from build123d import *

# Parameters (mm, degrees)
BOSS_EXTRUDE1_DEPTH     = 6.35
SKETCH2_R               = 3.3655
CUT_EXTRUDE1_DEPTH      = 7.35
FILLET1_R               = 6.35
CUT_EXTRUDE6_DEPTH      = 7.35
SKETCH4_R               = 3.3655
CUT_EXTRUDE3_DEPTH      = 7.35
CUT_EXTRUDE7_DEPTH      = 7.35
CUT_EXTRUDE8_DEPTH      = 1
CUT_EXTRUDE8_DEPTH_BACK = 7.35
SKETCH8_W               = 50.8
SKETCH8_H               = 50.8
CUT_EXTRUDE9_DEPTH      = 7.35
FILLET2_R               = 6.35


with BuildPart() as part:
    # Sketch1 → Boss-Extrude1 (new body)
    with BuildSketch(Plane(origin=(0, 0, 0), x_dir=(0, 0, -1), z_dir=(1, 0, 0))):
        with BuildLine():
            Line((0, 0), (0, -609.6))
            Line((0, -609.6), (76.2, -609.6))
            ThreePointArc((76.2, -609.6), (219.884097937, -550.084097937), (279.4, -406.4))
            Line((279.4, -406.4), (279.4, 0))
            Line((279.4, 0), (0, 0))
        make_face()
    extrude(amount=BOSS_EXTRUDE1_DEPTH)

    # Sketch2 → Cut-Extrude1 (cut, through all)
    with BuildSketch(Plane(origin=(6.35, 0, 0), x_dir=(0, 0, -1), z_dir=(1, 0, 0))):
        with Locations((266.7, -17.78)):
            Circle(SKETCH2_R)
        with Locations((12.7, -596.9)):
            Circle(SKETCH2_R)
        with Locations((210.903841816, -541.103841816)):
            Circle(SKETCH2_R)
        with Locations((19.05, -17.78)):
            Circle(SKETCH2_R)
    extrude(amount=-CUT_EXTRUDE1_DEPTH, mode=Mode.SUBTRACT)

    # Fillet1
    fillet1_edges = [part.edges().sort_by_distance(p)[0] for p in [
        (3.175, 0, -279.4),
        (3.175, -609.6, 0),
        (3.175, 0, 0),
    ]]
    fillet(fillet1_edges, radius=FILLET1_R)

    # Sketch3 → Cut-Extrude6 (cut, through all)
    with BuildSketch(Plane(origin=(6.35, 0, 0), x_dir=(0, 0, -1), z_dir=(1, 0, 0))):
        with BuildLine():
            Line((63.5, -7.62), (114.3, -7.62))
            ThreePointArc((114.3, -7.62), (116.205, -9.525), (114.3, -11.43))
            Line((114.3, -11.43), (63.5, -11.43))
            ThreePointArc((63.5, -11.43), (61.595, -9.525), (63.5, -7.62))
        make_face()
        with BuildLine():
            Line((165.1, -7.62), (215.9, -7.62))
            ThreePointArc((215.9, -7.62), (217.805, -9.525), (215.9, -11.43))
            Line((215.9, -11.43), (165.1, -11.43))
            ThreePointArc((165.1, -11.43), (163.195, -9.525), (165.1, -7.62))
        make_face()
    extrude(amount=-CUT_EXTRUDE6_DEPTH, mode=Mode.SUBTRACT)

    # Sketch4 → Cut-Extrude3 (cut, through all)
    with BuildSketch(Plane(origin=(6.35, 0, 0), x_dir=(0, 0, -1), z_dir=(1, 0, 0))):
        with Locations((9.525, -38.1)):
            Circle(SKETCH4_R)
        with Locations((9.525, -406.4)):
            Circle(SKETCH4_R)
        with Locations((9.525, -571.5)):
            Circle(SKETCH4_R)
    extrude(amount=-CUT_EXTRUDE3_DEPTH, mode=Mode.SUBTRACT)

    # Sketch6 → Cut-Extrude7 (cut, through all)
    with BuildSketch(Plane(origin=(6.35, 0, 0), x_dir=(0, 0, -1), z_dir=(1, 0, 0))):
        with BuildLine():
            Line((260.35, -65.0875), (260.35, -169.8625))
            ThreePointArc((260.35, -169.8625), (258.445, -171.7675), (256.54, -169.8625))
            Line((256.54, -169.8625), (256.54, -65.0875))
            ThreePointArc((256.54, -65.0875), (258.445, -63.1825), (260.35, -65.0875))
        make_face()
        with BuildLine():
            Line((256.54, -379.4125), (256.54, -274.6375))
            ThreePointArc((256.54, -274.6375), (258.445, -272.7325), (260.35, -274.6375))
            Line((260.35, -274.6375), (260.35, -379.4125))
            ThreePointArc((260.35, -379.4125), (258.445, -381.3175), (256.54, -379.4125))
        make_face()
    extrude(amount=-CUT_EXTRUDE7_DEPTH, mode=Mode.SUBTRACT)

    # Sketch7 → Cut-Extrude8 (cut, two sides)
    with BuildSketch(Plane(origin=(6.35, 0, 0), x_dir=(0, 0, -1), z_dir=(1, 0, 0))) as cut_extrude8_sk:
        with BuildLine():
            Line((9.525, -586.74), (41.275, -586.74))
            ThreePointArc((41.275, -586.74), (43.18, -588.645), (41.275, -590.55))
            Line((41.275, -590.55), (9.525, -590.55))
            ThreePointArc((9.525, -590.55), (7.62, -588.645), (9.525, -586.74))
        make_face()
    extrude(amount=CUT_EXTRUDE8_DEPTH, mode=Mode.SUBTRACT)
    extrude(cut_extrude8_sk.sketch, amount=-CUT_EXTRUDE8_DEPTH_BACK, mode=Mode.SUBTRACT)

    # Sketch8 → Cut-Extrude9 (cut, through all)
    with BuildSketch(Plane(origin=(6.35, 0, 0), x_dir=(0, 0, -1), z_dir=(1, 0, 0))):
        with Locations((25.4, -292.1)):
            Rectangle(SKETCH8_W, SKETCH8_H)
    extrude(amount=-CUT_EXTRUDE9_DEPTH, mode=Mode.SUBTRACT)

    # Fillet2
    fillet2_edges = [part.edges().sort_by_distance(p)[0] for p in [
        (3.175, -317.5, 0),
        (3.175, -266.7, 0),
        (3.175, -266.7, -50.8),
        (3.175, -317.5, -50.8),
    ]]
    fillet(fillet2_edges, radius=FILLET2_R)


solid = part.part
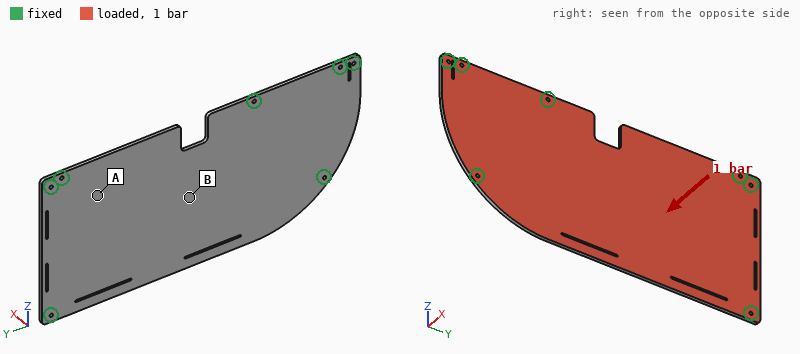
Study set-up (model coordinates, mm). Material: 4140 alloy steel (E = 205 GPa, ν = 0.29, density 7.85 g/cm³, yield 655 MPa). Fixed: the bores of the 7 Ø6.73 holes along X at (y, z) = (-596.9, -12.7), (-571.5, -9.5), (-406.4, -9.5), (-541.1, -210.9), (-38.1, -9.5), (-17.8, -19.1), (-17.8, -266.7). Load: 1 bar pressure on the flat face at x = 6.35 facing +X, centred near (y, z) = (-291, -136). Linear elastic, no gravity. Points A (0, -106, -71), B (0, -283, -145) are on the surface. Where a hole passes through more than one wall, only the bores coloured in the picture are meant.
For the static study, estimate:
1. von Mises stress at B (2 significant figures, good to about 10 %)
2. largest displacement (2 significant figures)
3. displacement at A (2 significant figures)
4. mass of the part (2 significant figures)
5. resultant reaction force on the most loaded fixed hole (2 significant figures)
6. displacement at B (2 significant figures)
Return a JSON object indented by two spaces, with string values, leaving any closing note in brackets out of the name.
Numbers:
{
  "von Mises stress at B": "120 MPa",
  "largest displacement": "5.6 mm",
  "displacement at A": "1.4 mm",
  "mass of the part": "7.8 kg",
  "resultant reaction force on the most loaded fixed hole": "4.9 kN",
  "displacement at B": "3.7 mm"
}
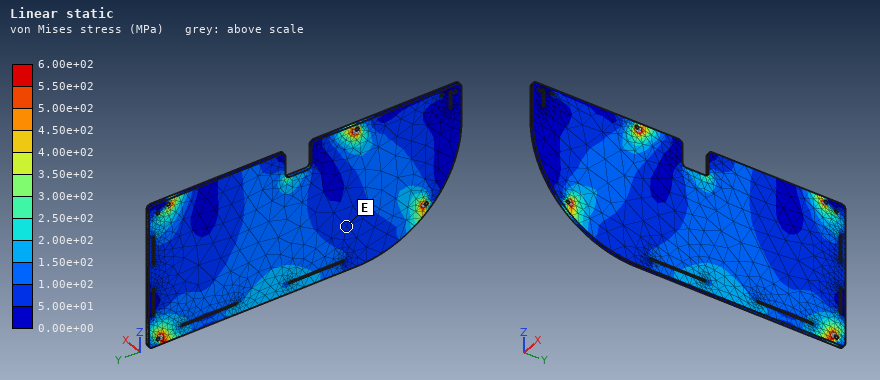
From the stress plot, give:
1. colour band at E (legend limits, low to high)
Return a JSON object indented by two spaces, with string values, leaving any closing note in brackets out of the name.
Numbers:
{
  "colour band at E": "5.00e+01 to 1.00e+02 MPa"
}
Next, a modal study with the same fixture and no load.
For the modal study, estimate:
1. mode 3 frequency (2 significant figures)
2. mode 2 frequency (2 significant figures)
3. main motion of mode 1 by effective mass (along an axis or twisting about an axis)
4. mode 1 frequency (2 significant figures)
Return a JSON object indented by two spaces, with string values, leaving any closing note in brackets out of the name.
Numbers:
{
  "mode 3 frequency": "330 Hz",
  "mode 2 frequency": "250 Hz",
  "main motion of mode 1 by effective mass": "along X",
  "mode 1 frequency": "130 Hz"
}
